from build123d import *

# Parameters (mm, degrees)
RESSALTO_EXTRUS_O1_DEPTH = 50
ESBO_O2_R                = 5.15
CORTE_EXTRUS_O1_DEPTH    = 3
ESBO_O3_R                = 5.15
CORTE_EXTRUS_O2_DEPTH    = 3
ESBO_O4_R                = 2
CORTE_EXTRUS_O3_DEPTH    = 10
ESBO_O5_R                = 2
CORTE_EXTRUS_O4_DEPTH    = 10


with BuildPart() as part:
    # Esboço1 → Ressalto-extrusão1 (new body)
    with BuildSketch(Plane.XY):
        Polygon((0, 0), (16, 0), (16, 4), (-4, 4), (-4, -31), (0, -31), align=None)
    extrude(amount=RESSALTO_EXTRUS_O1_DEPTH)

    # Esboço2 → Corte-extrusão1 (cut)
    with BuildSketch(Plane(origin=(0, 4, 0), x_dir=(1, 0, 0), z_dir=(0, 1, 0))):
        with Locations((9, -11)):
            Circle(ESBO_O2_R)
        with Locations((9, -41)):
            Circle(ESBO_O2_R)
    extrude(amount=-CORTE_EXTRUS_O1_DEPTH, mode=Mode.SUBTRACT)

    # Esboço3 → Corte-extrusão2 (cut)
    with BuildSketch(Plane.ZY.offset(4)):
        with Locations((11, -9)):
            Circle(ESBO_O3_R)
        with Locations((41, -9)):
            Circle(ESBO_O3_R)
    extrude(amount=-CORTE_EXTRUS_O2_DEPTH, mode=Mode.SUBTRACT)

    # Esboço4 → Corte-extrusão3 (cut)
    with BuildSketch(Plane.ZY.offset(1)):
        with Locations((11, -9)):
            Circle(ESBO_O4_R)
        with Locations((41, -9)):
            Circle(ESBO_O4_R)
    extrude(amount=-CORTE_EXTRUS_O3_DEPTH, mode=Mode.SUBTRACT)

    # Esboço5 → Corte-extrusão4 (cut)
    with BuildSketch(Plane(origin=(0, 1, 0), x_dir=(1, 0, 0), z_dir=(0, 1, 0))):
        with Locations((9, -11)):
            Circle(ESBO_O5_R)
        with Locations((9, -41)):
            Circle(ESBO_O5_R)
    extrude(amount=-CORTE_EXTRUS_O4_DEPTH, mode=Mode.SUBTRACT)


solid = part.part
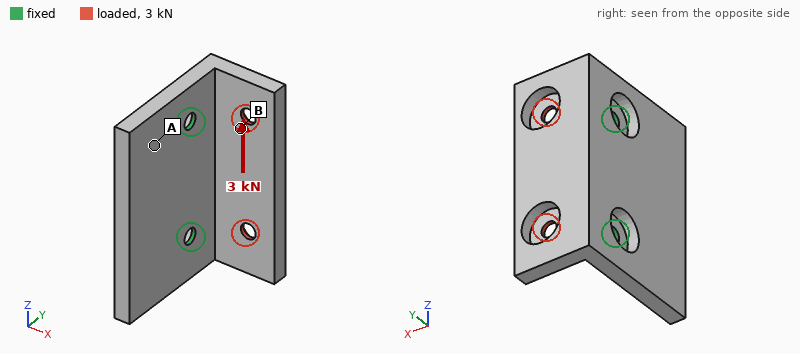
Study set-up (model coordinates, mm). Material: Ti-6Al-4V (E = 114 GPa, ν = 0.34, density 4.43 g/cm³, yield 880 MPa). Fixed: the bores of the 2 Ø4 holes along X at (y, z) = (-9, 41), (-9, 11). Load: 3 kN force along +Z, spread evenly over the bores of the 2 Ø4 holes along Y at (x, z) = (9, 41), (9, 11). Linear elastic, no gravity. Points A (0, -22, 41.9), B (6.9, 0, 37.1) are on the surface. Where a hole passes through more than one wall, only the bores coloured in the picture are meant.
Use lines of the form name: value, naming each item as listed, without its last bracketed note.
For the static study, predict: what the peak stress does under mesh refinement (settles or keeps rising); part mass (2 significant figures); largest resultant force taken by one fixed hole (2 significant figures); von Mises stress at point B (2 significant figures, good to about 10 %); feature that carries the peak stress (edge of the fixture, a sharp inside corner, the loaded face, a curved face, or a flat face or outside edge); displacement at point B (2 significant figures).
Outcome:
what the peak stress does under mesh refinement: keeps rising
part mass: 41 g
largest resultant force taken by one fixed hole: 2.0 kN
von Mises stress at point B: 140 MPa
feature that carries the peak stress: edge of the fixture
displacement at point B: 0.078 mm
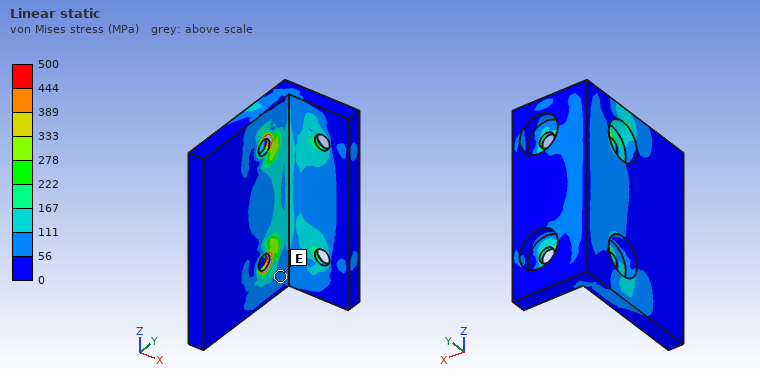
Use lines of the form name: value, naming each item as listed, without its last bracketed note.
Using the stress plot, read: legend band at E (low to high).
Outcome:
legend band at E: 56 to 111 MPa
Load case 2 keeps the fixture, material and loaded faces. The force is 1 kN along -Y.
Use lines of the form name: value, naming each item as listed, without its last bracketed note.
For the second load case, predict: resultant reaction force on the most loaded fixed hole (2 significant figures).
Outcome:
resultant reaction force on the most loaded fixed hole: 500 N
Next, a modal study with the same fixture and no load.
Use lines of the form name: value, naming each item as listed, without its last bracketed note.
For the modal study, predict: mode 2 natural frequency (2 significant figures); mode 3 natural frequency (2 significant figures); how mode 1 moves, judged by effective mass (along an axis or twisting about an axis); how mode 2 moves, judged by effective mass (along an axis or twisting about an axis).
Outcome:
mode 2 natural frequency: 5000 Hz
mode 3 natural frequency: 5500 Hz
how mode 1 moves, judged by effective mass: twisting about Z
how mode 2 moves, judged by effective mass: along X
